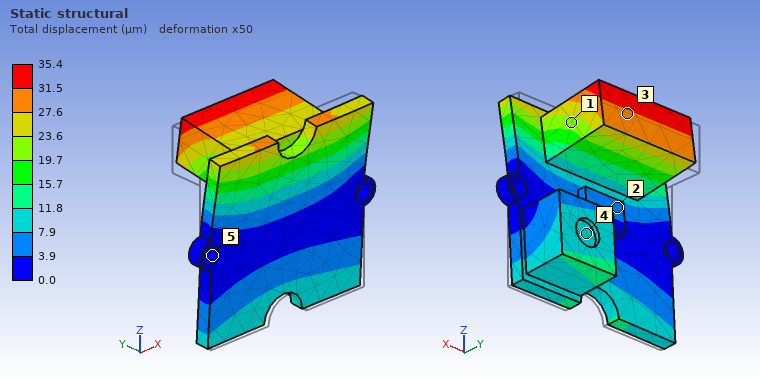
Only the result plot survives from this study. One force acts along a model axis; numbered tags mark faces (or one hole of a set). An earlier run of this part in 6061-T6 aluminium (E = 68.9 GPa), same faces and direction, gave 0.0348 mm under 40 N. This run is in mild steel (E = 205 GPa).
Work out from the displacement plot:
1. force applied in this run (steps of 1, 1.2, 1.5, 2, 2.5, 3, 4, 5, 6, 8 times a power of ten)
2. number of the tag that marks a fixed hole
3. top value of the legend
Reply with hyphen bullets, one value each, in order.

- 120 N
- 5
- 35.4 µm
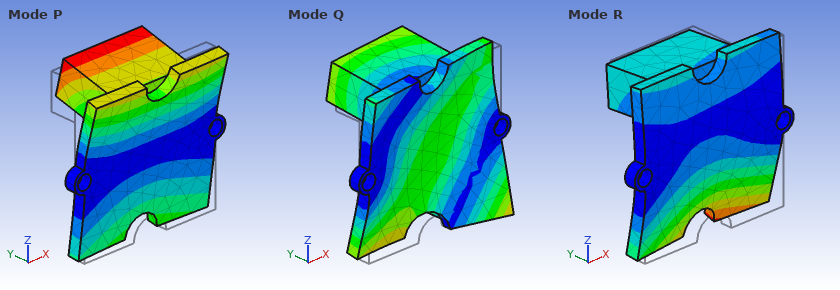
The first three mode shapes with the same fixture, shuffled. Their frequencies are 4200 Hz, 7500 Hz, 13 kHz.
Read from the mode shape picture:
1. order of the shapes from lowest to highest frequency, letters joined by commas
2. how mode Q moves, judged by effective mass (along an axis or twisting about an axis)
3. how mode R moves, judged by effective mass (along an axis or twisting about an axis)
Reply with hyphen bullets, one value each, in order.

- P, R, Q
- along Y
- along Y
